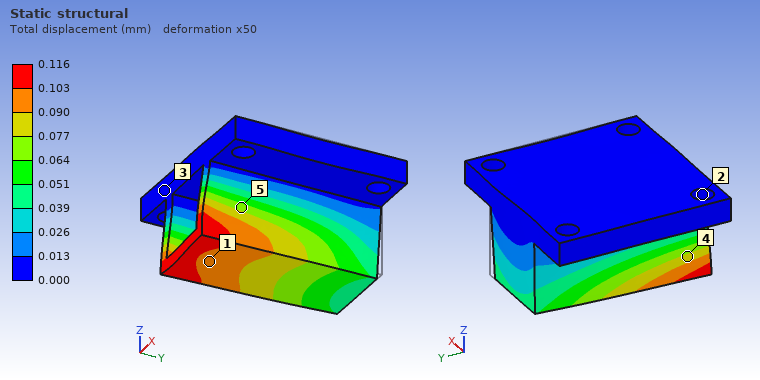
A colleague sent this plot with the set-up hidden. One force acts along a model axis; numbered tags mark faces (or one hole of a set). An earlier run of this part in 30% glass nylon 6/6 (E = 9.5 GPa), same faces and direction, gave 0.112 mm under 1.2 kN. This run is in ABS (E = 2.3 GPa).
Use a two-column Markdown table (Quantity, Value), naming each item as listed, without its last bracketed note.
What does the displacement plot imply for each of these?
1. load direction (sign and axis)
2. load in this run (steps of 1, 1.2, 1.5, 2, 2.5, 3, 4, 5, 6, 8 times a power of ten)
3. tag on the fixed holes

| Quantity | Value |
|---|---|
| load direction | -X |
| load in this run | 300 N |
| tag on the fixed holes | 2 |
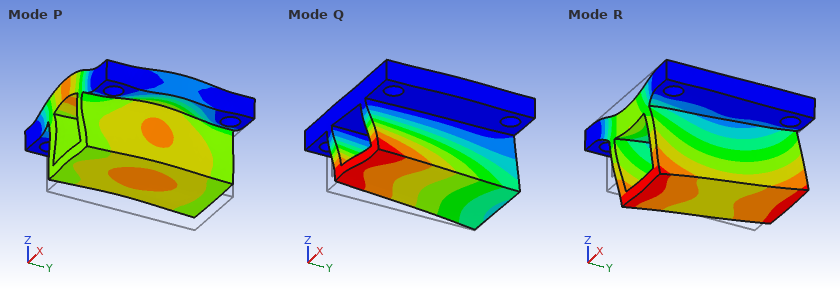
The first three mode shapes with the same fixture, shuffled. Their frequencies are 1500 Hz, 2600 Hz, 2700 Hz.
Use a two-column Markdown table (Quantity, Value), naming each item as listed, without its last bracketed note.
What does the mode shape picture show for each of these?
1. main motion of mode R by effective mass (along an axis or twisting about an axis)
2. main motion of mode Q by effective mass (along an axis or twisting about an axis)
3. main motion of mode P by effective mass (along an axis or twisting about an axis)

| Quantity | Value |
|---|---|
| main motion of mode R by effective mass | along Y |
| main motion of mode Q by effective mass | along X |
| main motion of mode P by effective mass | along Z |
